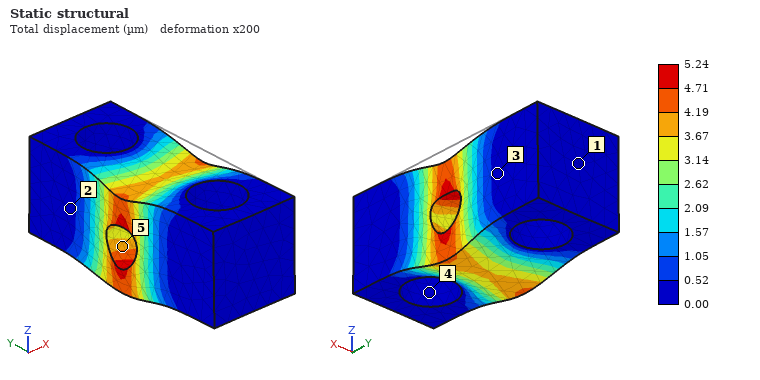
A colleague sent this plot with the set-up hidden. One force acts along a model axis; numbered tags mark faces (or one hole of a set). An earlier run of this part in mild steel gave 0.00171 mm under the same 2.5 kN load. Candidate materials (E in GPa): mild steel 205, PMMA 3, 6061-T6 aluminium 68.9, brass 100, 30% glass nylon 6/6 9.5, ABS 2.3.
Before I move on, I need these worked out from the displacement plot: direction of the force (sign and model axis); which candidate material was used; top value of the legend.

-Z
6061-T6 aluminium
5.24 µm
